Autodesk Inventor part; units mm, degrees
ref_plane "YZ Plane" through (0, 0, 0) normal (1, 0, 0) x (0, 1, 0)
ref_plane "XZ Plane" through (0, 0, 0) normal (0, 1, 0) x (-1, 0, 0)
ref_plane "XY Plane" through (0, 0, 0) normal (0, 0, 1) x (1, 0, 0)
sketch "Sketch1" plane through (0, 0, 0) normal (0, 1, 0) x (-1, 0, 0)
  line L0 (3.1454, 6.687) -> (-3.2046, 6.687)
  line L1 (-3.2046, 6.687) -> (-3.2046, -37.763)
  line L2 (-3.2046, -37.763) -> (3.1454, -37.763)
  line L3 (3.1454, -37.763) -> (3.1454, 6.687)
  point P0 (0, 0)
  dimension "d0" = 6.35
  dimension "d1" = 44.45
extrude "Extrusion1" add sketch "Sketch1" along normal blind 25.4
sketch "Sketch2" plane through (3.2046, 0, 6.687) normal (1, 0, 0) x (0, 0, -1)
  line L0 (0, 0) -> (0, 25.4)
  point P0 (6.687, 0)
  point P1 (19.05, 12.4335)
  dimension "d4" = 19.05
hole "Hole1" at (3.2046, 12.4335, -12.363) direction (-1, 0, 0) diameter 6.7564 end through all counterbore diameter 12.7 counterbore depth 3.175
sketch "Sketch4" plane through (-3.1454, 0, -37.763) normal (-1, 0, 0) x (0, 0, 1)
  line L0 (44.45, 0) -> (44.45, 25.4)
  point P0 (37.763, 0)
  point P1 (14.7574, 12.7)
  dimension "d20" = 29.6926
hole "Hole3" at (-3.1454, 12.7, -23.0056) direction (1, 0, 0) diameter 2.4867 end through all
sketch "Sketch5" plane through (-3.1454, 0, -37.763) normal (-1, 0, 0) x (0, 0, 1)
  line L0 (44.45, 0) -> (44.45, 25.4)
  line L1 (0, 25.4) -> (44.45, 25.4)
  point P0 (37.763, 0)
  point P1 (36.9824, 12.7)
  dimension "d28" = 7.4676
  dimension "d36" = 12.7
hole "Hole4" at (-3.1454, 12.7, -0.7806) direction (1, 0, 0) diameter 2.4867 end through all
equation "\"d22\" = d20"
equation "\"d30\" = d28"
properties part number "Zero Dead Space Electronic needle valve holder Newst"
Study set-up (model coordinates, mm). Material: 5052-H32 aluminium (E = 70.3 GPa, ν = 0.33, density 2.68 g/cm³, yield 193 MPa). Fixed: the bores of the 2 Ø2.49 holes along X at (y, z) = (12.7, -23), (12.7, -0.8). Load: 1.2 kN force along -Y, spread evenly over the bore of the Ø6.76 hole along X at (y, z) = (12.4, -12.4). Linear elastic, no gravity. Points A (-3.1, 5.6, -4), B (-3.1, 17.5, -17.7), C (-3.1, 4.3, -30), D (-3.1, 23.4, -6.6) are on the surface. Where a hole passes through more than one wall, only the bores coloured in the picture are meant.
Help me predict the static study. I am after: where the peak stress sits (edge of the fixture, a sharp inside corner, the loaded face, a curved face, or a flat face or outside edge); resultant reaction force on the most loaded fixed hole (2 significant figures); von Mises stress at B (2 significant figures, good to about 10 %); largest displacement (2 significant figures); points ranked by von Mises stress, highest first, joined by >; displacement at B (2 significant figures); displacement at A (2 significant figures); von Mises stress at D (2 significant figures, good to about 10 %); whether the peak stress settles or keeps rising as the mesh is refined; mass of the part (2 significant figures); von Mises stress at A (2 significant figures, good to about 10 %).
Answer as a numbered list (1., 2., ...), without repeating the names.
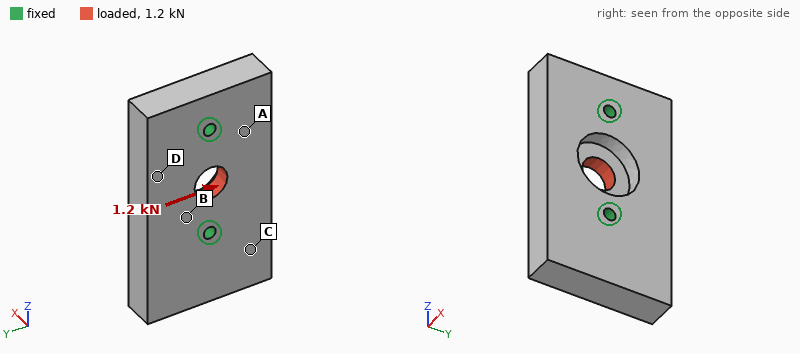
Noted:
1. edge of the fixture
2. 620 N
3. 14 MPa
4. 4.1 µm
5. B > A > D > C
6. 2.3 µm
7. 2.1 µm
8. 7.2 MPa
9. keeps rising
10. 18 g
11. 10 MPa
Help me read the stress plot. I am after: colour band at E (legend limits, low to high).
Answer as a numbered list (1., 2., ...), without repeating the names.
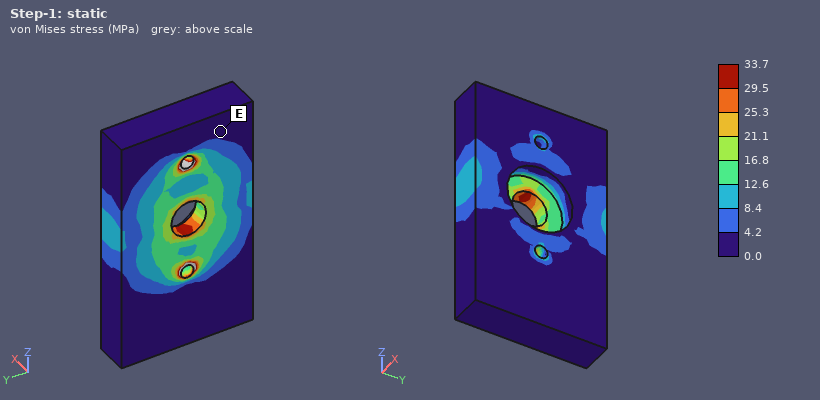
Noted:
1. 0.0 to 4.2 MPa
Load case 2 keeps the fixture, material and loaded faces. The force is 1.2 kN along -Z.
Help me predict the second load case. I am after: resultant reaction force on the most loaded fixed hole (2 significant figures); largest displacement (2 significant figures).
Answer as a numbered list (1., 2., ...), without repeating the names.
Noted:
1. 630 N
2. 2.4 µm
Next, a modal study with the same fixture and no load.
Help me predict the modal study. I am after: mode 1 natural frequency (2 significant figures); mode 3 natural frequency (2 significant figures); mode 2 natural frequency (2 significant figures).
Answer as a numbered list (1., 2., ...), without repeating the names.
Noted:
1. 16 kHz
2. 22 kHz
3. 16 kHz
